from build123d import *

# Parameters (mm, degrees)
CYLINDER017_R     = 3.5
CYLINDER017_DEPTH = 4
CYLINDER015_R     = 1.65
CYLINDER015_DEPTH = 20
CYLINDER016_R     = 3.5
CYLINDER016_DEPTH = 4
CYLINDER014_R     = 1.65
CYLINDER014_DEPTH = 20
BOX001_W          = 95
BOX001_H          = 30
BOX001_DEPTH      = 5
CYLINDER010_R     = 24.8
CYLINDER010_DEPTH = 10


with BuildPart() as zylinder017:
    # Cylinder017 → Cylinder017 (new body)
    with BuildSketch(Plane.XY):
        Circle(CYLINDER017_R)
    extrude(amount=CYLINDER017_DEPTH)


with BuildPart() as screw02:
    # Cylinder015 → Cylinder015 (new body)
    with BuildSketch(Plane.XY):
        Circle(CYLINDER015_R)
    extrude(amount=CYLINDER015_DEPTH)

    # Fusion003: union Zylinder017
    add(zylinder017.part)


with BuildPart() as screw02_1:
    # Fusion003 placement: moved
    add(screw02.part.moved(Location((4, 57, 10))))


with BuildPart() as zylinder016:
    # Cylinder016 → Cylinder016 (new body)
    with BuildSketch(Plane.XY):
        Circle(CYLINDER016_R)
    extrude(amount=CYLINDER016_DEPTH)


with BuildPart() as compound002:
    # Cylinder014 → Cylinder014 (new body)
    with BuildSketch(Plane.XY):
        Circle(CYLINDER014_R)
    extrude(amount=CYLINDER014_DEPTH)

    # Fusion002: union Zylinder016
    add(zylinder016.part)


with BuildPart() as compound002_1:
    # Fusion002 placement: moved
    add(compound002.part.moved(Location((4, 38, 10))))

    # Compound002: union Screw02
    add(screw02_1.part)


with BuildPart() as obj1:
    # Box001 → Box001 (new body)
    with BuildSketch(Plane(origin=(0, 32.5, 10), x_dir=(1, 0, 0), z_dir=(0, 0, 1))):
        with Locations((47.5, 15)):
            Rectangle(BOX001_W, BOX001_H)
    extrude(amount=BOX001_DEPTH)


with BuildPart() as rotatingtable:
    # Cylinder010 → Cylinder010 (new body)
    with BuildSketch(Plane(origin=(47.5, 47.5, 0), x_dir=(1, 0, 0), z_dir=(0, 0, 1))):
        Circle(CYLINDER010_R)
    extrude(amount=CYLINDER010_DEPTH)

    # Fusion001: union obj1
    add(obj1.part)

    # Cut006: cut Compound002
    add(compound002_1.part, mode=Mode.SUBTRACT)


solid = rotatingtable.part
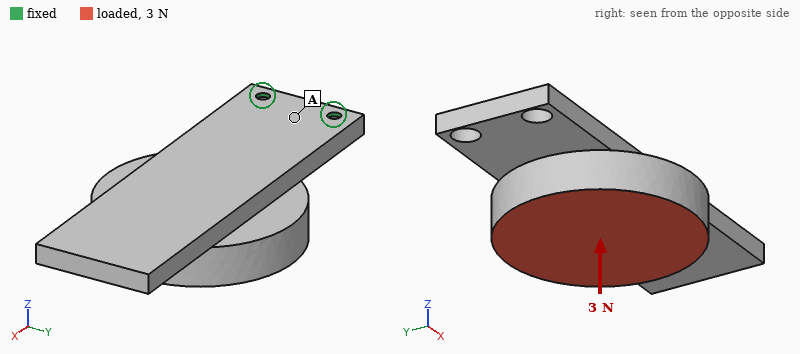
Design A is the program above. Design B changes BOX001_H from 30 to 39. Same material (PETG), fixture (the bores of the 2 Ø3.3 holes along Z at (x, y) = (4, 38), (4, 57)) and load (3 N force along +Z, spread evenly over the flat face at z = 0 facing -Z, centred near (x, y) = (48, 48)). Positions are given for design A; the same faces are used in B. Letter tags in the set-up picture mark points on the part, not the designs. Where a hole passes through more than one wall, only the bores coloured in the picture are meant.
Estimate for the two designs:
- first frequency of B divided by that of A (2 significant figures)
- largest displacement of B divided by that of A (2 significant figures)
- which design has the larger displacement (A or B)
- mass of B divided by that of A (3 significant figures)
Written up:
0.97
0.92
A
1.13
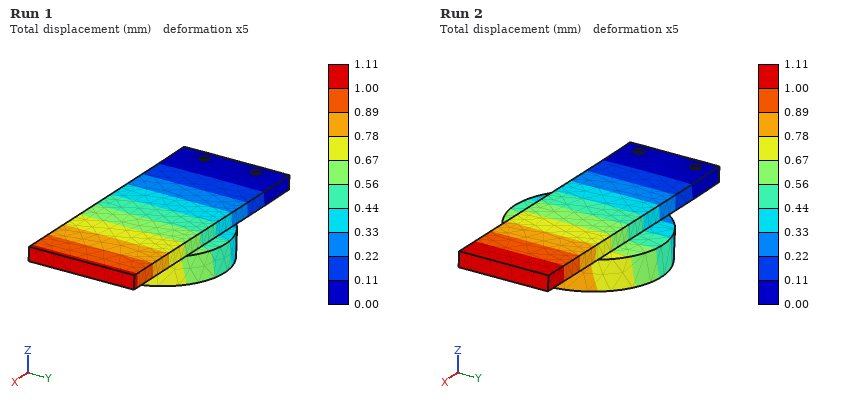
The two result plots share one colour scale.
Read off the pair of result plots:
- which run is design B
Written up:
Run 1
